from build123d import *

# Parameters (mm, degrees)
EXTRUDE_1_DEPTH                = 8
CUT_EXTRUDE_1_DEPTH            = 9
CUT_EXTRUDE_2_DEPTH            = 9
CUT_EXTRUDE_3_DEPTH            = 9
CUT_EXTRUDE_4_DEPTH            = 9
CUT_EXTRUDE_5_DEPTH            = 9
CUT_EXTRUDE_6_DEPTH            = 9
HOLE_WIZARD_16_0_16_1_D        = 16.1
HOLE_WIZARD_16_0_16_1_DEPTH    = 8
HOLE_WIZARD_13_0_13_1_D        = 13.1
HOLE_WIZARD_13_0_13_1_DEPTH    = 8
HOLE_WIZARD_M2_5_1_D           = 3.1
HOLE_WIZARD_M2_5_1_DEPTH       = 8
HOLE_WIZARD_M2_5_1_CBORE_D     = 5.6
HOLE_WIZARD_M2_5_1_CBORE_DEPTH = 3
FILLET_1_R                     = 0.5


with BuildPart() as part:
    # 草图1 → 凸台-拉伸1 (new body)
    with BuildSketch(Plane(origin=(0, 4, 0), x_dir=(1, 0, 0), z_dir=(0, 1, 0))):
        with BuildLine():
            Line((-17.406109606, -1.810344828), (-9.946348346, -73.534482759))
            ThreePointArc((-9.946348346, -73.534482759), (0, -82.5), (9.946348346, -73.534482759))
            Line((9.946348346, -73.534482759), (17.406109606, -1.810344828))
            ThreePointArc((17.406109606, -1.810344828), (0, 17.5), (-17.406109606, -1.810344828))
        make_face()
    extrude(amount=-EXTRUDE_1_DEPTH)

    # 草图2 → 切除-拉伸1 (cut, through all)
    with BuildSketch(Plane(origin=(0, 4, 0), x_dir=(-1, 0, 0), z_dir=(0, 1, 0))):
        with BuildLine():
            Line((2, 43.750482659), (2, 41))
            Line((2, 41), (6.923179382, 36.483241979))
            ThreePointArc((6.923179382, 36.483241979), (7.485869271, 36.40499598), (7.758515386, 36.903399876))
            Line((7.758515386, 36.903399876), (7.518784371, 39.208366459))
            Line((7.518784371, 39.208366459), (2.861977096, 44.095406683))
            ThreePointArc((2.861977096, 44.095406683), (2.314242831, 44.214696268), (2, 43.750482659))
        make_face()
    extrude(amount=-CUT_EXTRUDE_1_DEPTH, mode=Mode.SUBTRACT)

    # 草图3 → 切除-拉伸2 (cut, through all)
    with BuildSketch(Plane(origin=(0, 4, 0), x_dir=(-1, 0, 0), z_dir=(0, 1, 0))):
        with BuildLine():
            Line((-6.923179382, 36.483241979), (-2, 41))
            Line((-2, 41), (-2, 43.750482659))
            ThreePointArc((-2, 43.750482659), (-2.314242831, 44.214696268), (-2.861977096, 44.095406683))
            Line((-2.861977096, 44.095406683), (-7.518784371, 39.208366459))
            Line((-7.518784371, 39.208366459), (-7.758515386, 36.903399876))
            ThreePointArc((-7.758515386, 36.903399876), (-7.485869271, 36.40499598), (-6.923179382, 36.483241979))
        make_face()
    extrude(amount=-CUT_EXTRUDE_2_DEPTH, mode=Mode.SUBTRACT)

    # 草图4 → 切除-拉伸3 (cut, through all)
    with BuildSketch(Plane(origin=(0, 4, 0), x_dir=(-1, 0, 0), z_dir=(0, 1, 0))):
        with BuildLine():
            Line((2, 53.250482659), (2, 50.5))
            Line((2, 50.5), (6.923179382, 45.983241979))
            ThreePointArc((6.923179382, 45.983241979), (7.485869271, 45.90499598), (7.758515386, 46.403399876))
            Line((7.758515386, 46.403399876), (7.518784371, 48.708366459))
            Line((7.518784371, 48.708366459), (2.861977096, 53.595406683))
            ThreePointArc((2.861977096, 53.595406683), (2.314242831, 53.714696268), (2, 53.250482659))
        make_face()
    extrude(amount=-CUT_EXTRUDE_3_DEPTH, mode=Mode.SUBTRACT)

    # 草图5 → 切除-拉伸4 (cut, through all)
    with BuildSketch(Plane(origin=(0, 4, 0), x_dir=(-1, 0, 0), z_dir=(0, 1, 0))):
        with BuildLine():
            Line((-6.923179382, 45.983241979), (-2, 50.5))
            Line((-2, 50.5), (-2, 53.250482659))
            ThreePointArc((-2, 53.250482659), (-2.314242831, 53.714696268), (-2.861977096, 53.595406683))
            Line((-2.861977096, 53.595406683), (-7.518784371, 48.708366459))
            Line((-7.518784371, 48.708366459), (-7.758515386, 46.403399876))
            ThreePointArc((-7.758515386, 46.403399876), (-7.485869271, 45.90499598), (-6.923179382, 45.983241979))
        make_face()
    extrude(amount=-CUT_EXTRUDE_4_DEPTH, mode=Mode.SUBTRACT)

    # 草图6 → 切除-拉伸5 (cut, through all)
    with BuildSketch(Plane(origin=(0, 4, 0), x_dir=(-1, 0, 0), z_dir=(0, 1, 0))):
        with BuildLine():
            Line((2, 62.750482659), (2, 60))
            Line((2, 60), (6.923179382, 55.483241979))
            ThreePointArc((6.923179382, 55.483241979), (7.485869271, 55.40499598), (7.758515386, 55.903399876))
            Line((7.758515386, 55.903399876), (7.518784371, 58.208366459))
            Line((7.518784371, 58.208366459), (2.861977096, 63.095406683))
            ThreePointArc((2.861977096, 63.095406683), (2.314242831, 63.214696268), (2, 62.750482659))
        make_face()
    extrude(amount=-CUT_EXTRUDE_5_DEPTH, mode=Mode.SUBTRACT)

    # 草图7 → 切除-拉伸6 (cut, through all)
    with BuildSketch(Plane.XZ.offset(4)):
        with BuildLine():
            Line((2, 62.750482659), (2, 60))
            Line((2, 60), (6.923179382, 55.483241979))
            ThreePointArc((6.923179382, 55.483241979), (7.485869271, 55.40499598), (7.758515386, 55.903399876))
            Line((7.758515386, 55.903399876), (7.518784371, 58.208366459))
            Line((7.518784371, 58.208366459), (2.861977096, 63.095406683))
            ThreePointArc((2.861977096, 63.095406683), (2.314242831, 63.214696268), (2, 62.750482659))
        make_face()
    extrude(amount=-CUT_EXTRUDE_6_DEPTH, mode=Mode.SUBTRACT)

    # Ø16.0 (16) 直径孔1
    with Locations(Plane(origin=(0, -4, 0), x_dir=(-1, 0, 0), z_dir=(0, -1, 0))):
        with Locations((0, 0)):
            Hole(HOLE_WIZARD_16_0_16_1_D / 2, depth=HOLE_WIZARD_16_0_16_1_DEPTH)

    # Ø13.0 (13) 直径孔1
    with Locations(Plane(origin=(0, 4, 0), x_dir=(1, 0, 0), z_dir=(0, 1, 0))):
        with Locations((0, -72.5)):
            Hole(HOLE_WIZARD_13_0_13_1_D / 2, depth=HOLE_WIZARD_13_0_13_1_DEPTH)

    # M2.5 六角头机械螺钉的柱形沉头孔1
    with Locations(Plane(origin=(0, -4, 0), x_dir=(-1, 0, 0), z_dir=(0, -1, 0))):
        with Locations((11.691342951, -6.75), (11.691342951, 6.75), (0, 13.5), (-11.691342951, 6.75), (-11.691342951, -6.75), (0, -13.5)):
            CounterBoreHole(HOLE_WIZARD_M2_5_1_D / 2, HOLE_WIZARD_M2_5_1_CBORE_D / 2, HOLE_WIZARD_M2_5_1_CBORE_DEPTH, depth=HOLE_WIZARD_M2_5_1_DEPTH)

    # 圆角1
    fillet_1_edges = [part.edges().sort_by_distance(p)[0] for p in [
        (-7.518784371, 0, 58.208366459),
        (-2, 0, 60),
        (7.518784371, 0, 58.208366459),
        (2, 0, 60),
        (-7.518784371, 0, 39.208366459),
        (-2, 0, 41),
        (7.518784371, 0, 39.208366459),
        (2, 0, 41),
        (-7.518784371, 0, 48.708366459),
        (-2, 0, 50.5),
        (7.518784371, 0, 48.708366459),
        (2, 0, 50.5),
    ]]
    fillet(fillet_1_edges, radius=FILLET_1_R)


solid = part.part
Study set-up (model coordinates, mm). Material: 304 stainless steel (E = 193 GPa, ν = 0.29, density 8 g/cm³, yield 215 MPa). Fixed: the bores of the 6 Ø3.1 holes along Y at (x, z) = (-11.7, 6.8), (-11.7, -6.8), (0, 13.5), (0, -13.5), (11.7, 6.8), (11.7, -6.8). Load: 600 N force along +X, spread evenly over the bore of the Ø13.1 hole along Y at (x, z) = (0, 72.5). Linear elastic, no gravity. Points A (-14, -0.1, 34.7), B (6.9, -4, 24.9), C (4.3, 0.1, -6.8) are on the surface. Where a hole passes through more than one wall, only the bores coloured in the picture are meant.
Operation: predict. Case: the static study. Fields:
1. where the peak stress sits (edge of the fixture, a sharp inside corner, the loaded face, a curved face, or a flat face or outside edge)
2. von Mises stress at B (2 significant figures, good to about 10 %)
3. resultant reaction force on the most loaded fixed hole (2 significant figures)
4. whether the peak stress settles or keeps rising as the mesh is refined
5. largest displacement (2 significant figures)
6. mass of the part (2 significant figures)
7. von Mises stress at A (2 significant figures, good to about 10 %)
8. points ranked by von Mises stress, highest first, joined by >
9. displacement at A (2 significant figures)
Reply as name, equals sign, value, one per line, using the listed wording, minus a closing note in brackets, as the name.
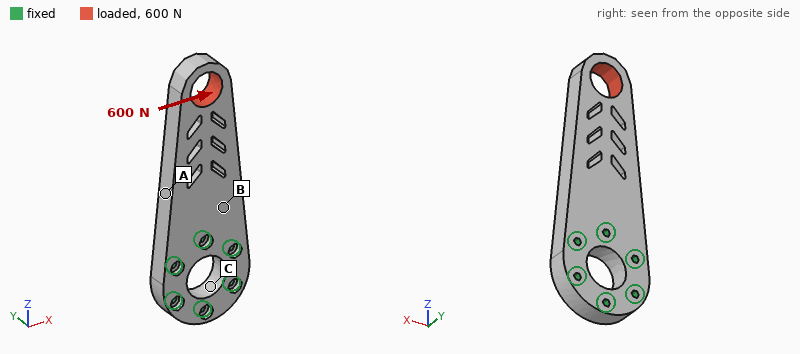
where the peak stress sits = edge of the fixture
von Mises stress at B = 9.3 MPa
resultant reaction force on the most loaded fixed hole = 1.2 kN
whether the peak stress settles or keeps rising as the mesh is refined = keeps rising
largest displacement = 31 µm
mass of the part = 130 g
von Mises stress at A = 27 MPa
points ranked by von Mises stress, highest first, joined by > = A > B > C
displacement at A = 5.9 µm
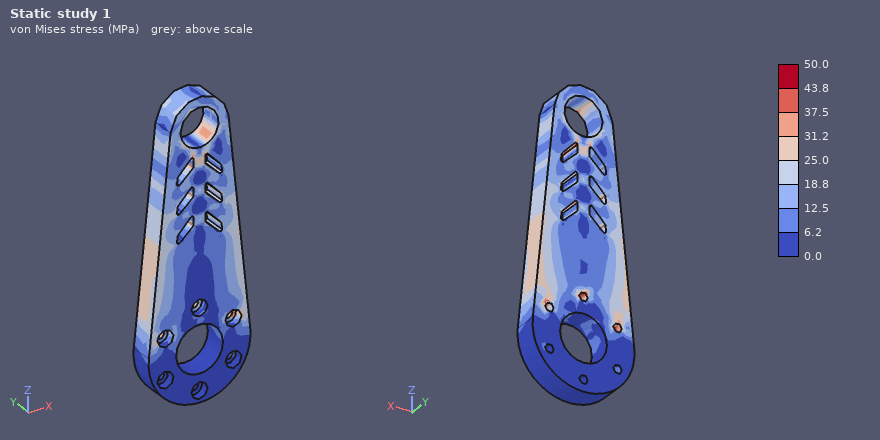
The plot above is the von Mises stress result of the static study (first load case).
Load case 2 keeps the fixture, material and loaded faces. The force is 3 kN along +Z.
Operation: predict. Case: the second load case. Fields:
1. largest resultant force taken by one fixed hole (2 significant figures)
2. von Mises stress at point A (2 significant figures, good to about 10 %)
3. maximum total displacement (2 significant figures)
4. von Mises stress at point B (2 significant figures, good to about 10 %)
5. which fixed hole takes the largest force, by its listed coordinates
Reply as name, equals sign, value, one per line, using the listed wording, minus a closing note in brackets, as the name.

largest resultant force taken by one fixed hole = 1.2 kN
von Mises stress at point A = 17 MPa
maximum total displacement = 13 µm
von Mises stress at point B = 12 MPa
which fixed hole takes the largest force, by its listed coordinates = (0, 13.5)
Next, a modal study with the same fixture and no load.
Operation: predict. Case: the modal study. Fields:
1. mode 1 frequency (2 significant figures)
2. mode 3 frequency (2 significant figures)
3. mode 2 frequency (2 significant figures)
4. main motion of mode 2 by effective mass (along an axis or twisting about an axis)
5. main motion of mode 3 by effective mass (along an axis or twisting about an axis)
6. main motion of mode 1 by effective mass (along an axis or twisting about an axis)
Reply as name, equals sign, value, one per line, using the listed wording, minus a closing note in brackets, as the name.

mode 1 frequency = 1700 Hz
mode 3 frequency = 6900 Hz
mode 2 frequency = 5200 Hz
main motion of mode 2 by effective mass = along X
main motion of mode 3 by effective mass = twisting about Z
main motion of mode 1 by effective mass = along Y
